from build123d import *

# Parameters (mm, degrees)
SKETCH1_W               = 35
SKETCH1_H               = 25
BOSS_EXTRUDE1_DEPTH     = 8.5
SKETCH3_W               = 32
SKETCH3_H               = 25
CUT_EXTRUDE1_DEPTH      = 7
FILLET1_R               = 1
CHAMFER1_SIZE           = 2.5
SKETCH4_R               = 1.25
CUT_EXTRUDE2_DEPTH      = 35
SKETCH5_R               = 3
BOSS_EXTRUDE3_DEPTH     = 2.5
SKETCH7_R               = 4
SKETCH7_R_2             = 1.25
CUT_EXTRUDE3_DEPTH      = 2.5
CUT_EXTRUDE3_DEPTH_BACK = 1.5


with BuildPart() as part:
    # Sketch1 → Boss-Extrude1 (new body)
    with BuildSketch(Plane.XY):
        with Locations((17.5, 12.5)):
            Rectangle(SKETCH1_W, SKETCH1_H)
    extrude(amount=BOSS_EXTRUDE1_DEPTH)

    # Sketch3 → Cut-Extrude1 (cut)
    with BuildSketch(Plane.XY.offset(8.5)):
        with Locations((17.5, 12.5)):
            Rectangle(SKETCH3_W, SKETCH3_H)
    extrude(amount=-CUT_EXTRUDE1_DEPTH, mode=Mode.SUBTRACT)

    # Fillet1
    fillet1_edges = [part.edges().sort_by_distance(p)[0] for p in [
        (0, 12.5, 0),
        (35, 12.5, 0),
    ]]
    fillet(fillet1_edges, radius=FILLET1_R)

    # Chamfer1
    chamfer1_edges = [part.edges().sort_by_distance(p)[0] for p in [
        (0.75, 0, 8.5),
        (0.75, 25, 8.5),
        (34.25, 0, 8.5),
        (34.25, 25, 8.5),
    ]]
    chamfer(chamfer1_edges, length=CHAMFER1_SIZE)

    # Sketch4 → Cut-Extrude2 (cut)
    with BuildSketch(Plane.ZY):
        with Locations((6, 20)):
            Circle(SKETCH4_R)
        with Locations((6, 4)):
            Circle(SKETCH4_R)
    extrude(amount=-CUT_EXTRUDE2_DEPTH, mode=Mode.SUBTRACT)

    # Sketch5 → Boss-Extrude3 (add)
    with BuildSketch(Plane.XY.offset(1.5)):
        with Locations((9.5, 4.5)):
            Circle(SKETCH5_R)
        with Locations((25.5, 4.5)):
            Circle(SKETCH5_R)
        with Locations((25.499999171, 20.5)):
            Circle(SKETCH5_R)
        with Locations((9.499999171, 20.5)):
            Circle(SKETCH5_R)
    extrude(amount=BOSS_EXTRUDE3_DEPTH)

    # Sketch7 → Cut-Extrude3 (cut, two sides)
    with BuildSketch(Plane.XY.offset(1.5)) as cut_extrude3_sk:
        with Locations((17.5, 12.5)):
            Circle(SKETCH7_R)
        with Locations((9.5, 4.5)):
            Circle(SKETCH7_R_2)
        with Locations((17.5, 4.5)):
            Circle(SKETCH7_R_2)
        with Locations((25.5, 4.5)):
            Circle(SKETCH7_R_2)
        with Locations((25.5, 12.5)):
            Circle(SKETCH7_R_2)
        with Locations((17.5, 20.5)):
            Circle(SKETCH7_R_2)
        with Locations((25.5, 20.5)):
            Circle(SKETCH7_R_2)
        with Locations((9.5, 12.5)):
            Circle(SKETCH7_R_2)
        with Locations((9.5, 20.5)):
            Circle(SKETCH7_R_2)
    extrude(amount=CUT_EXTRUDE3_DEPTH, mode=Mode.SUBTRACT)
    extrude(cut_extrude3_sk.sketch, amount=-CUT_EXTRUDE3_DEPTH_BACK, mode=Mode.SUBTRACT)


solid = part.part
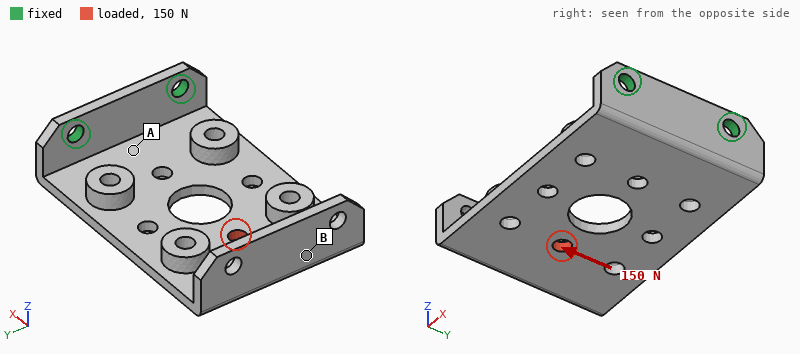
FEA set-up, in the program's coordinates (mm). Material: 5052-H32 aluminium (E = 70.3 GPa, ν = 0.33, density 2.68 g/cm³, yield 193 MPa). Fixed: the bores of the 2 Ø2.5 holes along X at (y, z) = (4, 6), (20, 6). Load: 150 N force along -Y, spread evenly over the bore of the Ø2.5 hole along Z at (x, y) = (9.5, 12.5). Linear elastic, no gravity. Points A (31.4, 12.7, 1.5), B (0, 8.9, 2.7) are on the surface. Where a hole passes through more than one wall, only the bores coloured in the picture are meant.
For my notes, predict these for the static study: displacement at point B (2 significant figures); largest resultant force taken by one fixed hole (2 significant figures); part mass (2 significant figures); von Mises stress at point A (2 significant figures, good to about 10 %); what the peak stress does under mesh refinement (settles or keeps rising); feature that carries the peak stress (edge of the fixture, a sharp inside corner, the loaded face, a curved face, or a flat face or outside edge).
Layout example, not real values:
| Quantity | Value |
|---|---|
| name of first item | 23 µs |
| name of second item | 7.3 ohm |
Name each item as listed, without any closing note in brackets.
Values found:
| Quantity | Value |
|---|---|
| displacement at point B | 0.14 mm |
| largest resultant force taken by one fixed hole | 230 N |
| part mass | 5.0 g |
| von Mises stress at point A | 46 MPa |
| what the peak stress does under mesh refinement | keeps rising |
| feature that carries the peak stress | edge of the fixture |
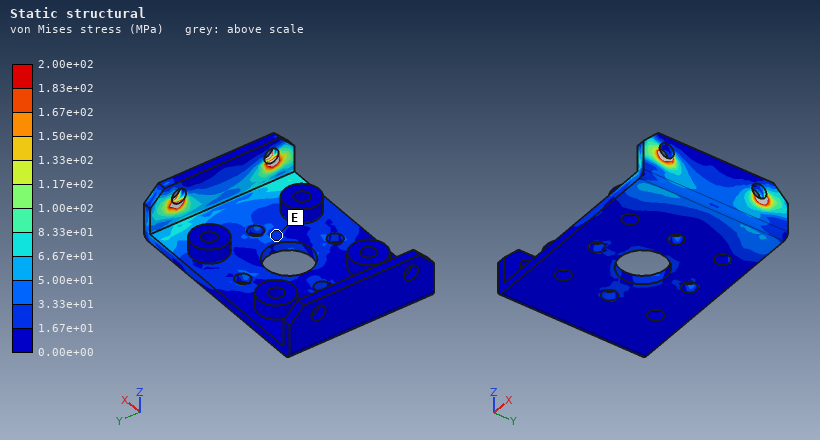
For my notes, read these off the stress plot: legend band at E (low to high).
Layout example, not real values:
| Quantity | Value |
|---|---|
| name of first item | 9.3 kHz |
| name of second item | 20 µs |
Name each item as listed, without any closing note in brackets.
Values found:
| Quantity | Value |
|---|---|
| legend band at E | 1.67e+01 to 3.33e+01 MPa |
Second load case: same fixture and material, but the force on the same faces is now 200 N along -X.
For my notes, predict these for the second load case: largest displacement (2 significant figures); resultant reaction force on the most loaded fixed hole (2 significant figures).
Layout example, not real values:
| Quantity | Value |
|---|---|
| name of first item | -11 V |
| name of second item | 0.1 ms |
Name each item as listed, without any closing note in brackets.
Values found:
| Quantity | Value |
|---|---|
| largest displacement | 0.19 mm |
| resultant reaction force on the most loaded fixed hole | 110 N |
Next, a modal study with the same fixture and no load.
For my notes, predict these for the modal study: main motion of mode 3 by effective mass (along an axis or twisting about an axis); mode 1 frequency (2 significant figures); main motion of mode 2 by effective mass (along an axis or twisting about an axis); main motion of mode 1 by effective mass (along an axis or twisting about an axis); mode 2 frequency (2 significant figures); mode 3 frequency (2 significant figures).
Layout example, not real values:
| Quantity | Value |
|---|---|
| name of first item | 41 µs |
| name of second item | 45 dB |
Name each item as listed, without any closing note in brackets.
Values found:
| Quantity | Value |
|---|---|
| main motion of mode 3 by effective mass | along Y |
| mode 1 frequency | 670 Hz |
| main motion of mode 2 by effective mass | along Y |
| main motion of mode 1 by effective mass | along Z |
| mode 2 frequency | 2200 Hz |
| mode 3 frequency | 3700 Hz |
